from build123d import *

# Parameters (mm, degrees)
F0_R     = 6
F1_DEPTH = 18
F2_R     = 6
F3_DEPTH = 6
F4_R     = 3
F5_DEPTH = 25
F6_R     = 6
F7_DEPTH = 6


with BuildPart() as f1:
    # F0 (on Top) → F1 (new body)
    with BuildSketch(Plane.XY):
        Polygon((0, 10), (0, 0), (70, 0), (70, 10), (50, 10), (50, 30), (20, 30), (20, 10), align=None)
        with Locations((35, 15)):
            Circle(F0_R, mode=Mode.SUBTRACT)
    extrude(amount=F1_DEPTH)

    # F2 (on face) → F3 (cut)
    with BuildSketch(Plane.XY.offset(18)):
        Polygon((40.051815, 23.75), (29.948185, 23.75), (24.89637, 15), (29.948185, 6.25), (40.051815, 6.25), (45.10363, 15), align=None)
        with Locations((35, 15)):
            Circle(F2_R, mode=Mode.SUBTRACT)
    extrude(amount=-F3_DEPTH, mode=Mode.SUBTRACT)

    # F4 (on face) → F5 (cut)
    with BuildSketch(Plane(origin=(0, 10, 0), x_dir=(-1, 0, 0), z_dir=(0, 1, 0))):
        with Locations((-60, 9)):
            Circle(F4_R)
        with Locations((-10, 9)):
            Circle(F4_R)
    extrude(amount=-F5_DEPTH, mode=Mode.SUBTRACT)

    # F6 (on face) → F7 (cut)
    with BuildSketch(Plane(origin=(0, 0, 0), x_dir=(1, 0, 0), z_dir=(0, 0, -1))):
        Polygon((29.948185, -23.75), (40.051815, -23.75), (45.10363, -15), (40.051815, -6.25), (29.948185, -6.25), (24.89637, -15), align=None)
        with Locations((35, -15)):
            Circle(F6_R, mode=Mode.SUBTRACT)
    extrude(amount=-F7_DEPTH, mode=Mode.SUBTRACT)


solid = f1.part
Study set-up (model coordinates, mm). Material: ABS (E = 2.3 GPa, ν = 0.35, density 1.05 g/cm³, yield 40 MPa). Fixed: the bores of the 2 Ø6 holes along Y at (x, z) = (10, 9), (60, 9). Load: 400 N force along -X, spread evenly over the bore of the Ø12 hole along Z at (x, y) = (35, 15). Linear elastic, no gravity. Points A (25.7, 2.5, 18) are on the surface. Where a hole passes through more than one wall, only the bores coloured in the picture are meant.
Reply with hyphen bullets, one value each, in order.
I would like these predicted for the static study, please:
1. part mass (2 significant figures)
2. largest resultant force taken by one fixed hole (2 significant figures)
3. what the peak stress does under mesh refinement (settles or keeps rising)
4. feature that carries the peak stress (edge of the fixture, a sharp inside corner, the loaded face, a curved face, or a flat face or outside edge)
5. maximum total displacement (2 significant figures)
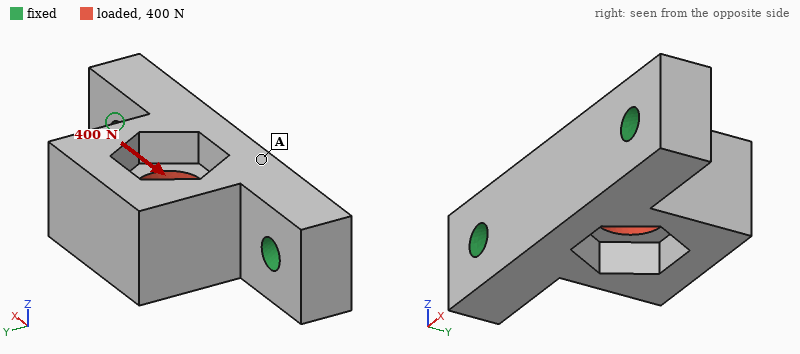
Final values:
- 20 g
- 220 N
- keeps rising
- edge of the fixture
- 49 µm
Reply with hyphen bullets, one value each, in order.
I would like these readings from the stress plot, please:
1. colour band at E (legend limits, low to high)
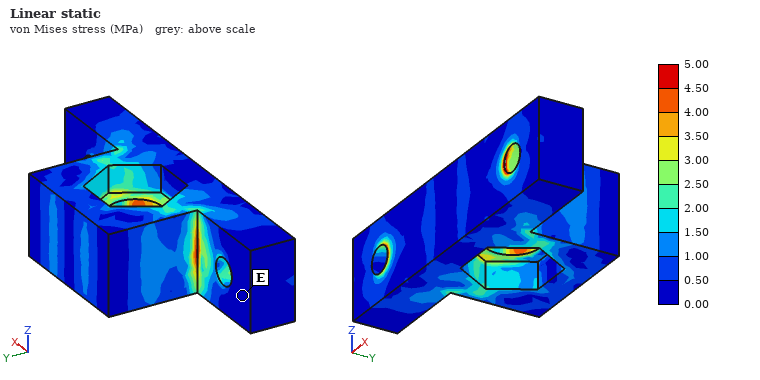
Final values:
- 0.00 to 0.50 MPa
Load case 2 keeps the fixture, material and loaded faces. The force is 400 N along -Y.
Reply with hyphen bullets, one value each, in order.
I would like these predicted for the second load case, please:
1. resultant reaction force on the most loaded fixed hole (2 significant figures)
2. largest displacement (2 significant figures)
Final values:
- 200 N
- 55 µm
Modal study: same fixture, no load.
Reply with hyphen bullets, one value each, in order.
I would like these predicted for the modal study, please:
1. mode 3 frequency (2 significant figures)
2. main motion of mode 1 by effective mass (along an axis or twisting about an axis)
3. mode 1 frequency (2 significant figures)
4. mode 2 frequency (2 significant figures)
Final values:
- 4400 Hz
- along Z
- 2100 Hz
- 4200 Hz
